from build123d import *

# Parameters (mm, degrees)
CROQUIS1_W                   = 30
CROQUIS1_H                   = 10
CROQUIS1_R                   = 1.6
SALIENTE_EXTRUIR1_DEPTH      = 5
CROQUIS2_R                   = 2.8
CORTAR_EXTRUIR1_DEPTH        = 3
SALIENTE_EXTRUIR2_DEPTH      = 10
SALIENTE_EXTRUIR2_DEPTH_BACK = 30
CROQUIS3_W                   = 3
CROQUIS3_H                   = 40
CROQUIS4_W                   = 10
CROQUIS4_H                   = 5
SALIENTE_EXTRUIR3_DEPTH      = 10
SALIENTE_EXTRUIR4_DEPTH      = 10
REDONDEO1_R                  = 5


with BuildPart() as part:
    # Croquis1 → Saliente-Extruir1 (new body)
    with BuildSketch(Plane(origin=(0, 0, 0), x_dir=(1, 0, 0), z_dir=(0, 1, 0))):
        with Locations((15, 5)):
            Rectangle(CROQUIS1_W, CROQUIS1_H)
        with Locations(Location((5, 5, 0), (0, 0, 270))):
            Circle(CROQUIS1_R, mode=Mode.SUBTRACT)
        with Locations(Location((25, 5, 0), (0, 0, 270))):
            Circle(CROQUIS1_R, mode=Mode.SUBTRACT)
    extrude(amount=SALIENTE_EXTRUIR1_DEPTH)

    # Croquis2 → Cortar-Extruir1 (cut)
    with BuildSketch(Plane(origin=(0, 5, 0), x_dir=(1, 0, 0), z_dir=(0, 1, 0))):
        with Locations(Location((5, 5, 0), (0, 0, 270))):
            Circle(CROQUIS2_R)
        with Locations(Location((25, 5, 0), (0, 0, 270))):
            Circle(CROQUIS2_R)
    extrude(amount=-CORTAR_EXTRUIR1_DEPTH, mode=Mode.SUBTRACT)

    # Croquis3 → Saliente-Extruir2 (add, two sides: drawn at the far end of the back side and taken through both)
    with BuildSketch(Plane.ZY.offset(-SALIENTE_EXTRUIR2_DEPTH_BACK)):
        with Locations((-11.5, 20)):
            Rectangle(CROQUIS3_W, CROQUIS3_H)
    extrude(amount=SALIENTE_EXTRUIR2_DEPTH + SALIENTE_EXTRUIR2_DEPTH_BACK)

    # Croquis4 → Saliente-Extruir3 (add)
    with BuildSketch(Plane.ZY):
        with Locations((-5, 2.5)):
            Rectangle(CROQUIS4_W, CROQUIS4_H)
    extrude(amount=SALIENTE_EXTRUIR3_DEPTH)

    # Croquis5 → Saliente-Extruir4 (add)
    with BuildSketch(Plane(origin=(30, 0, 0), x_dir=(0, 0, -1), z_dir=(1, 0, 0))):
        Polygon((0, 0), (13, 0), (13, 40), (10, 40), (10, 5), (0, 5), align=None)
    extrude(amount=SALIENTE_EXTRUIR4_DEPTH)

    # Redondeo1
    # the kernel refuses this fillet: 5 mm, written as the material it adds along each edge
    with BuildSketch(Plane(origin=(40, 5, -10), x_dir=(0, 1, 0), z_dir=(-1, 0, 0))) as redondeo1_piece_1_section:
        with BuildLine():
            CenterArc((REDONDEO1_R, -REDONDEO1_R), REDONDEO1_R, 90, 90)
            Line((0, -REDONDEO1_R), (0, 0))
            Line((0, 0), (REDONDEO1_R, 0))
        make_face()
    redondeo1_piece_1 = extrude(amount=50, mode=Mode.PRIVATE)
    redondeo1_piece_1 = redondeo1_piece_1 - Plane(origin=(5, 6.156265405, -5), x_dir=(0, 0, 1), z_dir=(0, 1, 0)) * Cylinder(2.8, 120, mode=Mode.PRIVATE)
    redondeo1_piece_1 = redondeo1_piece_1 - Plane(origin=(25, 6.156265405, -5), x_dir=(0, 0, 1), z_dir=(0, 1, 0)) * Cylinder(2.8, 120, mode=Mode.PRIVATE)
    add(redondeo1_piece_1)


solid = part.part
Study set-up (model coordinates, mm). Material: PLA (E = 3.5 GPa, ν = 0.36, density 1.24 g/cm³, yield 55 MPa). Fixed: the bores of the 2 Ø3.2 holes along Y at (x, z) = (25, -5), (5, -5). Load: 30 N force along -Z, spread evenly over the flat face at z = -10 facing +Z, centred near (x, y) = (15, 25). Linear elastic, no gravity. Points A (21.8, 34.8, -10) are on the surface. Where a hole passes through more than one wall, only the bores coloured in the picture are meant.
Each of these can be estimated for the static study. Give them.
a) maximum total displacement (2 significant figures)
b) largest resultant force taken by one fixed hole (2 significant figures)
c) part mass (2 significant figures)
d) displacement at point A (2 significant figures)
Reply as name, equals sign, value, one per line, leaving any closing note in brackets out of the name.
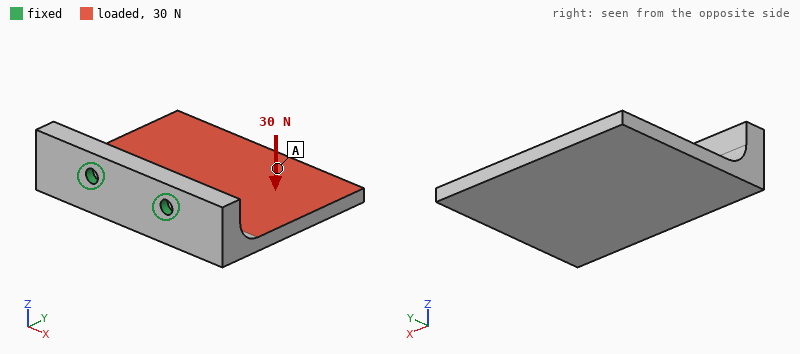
maximum total displacement = 0.75 mm
largest resultant force taken by one fixed hole = 15 N
part mass = 11 g
displacement at point A = 0.61 mm
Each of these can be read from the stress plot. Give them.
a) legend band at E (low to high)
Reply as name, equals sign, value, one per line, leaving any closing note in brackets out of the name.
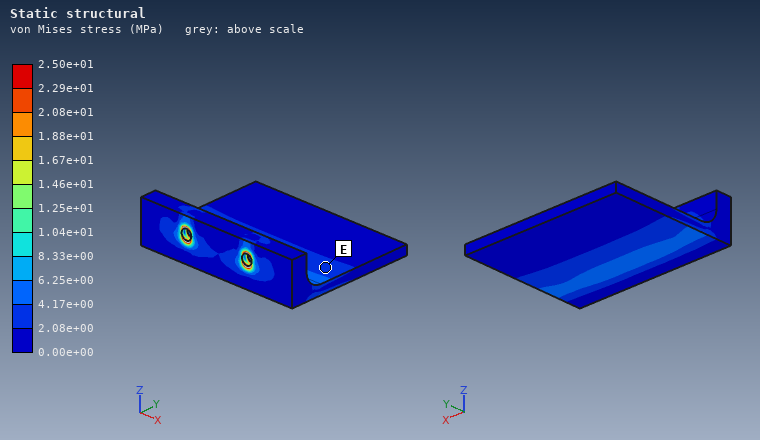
legend band at E = 2.08e+00 to 4.17e+00 MPa
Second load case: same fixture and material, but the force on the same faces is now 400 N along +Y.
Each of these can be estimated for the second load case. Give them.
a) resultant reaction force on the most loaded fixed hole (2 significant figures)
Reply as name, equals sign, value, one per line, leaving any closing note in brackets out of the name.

resultant reaction force on the most loaded fixed hole = 200 N
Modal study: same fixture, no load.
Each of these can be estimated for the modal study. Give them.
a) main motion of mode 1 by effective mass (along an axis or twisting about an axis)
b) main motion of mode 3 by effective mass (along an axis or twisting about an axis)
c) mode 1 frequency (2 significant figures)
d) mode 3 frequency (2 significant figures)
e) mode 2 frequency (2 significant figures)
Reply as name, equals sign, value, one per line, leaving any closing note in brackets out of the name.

main motion of mode 1 by effective mass = along Z
main motion of mode 3 by effective mass = along X
mode 1 frequency = 520 Hz
mode 3 frequency = 1800 Hz
mode 2 frequency = 1100 Hz
